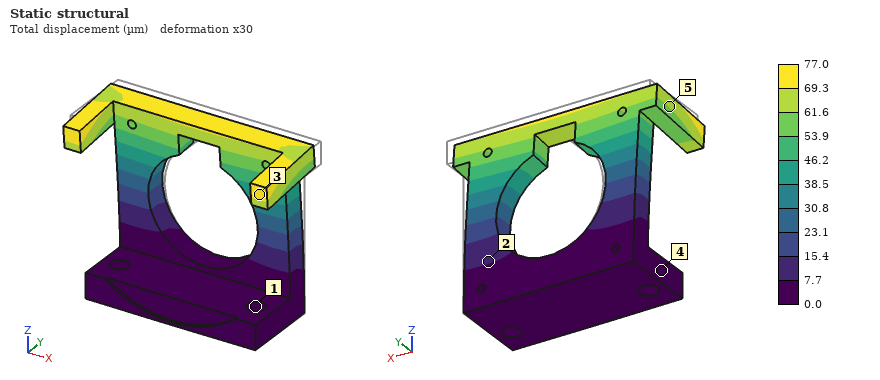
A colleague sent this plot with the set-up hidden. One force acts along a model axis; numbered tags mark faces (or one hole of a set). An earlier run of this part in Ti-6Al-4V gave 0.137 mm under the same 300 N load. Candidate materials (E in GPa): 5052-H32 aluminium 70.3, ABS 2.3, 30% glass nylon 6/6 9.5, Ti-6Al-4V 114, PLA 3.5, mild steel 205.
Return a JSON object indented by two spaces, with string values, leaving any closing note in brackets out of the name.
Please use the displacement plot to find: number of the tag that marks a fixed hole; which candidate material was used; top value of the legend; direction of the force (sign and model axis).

{
  "number of the tag that marks a fixed hole": "1",
  "which candidate material was used": "mild steel",
  "top value of the legend": "77.0 µm",
  "direction of the force": "-Y"
}
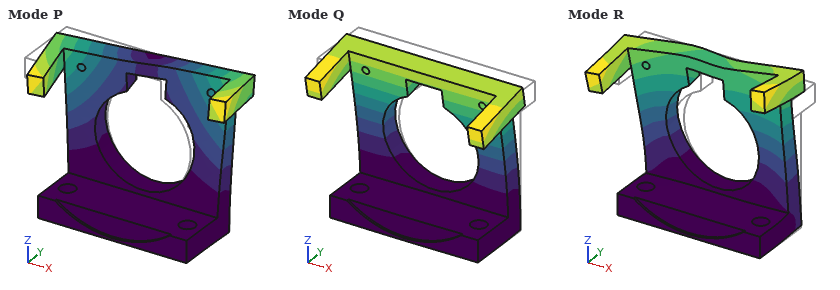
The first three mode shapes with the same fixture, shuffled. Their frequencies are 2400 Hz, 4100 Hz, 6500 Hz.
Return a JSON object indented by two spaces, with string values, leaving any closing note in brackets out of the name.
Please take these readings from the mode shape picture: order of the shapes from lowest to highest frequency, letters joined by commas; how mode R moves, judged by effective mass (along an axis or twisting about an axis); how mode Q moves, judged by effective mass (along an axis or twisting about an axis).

{
  "order of the shapes from lowest to highest frequency, letters joined by commas": "Q, P, R",
  "how mode R moves, judged by effective mass": "along X",
  "how mode Q moves, judged by effective mass": "along Y"
}
